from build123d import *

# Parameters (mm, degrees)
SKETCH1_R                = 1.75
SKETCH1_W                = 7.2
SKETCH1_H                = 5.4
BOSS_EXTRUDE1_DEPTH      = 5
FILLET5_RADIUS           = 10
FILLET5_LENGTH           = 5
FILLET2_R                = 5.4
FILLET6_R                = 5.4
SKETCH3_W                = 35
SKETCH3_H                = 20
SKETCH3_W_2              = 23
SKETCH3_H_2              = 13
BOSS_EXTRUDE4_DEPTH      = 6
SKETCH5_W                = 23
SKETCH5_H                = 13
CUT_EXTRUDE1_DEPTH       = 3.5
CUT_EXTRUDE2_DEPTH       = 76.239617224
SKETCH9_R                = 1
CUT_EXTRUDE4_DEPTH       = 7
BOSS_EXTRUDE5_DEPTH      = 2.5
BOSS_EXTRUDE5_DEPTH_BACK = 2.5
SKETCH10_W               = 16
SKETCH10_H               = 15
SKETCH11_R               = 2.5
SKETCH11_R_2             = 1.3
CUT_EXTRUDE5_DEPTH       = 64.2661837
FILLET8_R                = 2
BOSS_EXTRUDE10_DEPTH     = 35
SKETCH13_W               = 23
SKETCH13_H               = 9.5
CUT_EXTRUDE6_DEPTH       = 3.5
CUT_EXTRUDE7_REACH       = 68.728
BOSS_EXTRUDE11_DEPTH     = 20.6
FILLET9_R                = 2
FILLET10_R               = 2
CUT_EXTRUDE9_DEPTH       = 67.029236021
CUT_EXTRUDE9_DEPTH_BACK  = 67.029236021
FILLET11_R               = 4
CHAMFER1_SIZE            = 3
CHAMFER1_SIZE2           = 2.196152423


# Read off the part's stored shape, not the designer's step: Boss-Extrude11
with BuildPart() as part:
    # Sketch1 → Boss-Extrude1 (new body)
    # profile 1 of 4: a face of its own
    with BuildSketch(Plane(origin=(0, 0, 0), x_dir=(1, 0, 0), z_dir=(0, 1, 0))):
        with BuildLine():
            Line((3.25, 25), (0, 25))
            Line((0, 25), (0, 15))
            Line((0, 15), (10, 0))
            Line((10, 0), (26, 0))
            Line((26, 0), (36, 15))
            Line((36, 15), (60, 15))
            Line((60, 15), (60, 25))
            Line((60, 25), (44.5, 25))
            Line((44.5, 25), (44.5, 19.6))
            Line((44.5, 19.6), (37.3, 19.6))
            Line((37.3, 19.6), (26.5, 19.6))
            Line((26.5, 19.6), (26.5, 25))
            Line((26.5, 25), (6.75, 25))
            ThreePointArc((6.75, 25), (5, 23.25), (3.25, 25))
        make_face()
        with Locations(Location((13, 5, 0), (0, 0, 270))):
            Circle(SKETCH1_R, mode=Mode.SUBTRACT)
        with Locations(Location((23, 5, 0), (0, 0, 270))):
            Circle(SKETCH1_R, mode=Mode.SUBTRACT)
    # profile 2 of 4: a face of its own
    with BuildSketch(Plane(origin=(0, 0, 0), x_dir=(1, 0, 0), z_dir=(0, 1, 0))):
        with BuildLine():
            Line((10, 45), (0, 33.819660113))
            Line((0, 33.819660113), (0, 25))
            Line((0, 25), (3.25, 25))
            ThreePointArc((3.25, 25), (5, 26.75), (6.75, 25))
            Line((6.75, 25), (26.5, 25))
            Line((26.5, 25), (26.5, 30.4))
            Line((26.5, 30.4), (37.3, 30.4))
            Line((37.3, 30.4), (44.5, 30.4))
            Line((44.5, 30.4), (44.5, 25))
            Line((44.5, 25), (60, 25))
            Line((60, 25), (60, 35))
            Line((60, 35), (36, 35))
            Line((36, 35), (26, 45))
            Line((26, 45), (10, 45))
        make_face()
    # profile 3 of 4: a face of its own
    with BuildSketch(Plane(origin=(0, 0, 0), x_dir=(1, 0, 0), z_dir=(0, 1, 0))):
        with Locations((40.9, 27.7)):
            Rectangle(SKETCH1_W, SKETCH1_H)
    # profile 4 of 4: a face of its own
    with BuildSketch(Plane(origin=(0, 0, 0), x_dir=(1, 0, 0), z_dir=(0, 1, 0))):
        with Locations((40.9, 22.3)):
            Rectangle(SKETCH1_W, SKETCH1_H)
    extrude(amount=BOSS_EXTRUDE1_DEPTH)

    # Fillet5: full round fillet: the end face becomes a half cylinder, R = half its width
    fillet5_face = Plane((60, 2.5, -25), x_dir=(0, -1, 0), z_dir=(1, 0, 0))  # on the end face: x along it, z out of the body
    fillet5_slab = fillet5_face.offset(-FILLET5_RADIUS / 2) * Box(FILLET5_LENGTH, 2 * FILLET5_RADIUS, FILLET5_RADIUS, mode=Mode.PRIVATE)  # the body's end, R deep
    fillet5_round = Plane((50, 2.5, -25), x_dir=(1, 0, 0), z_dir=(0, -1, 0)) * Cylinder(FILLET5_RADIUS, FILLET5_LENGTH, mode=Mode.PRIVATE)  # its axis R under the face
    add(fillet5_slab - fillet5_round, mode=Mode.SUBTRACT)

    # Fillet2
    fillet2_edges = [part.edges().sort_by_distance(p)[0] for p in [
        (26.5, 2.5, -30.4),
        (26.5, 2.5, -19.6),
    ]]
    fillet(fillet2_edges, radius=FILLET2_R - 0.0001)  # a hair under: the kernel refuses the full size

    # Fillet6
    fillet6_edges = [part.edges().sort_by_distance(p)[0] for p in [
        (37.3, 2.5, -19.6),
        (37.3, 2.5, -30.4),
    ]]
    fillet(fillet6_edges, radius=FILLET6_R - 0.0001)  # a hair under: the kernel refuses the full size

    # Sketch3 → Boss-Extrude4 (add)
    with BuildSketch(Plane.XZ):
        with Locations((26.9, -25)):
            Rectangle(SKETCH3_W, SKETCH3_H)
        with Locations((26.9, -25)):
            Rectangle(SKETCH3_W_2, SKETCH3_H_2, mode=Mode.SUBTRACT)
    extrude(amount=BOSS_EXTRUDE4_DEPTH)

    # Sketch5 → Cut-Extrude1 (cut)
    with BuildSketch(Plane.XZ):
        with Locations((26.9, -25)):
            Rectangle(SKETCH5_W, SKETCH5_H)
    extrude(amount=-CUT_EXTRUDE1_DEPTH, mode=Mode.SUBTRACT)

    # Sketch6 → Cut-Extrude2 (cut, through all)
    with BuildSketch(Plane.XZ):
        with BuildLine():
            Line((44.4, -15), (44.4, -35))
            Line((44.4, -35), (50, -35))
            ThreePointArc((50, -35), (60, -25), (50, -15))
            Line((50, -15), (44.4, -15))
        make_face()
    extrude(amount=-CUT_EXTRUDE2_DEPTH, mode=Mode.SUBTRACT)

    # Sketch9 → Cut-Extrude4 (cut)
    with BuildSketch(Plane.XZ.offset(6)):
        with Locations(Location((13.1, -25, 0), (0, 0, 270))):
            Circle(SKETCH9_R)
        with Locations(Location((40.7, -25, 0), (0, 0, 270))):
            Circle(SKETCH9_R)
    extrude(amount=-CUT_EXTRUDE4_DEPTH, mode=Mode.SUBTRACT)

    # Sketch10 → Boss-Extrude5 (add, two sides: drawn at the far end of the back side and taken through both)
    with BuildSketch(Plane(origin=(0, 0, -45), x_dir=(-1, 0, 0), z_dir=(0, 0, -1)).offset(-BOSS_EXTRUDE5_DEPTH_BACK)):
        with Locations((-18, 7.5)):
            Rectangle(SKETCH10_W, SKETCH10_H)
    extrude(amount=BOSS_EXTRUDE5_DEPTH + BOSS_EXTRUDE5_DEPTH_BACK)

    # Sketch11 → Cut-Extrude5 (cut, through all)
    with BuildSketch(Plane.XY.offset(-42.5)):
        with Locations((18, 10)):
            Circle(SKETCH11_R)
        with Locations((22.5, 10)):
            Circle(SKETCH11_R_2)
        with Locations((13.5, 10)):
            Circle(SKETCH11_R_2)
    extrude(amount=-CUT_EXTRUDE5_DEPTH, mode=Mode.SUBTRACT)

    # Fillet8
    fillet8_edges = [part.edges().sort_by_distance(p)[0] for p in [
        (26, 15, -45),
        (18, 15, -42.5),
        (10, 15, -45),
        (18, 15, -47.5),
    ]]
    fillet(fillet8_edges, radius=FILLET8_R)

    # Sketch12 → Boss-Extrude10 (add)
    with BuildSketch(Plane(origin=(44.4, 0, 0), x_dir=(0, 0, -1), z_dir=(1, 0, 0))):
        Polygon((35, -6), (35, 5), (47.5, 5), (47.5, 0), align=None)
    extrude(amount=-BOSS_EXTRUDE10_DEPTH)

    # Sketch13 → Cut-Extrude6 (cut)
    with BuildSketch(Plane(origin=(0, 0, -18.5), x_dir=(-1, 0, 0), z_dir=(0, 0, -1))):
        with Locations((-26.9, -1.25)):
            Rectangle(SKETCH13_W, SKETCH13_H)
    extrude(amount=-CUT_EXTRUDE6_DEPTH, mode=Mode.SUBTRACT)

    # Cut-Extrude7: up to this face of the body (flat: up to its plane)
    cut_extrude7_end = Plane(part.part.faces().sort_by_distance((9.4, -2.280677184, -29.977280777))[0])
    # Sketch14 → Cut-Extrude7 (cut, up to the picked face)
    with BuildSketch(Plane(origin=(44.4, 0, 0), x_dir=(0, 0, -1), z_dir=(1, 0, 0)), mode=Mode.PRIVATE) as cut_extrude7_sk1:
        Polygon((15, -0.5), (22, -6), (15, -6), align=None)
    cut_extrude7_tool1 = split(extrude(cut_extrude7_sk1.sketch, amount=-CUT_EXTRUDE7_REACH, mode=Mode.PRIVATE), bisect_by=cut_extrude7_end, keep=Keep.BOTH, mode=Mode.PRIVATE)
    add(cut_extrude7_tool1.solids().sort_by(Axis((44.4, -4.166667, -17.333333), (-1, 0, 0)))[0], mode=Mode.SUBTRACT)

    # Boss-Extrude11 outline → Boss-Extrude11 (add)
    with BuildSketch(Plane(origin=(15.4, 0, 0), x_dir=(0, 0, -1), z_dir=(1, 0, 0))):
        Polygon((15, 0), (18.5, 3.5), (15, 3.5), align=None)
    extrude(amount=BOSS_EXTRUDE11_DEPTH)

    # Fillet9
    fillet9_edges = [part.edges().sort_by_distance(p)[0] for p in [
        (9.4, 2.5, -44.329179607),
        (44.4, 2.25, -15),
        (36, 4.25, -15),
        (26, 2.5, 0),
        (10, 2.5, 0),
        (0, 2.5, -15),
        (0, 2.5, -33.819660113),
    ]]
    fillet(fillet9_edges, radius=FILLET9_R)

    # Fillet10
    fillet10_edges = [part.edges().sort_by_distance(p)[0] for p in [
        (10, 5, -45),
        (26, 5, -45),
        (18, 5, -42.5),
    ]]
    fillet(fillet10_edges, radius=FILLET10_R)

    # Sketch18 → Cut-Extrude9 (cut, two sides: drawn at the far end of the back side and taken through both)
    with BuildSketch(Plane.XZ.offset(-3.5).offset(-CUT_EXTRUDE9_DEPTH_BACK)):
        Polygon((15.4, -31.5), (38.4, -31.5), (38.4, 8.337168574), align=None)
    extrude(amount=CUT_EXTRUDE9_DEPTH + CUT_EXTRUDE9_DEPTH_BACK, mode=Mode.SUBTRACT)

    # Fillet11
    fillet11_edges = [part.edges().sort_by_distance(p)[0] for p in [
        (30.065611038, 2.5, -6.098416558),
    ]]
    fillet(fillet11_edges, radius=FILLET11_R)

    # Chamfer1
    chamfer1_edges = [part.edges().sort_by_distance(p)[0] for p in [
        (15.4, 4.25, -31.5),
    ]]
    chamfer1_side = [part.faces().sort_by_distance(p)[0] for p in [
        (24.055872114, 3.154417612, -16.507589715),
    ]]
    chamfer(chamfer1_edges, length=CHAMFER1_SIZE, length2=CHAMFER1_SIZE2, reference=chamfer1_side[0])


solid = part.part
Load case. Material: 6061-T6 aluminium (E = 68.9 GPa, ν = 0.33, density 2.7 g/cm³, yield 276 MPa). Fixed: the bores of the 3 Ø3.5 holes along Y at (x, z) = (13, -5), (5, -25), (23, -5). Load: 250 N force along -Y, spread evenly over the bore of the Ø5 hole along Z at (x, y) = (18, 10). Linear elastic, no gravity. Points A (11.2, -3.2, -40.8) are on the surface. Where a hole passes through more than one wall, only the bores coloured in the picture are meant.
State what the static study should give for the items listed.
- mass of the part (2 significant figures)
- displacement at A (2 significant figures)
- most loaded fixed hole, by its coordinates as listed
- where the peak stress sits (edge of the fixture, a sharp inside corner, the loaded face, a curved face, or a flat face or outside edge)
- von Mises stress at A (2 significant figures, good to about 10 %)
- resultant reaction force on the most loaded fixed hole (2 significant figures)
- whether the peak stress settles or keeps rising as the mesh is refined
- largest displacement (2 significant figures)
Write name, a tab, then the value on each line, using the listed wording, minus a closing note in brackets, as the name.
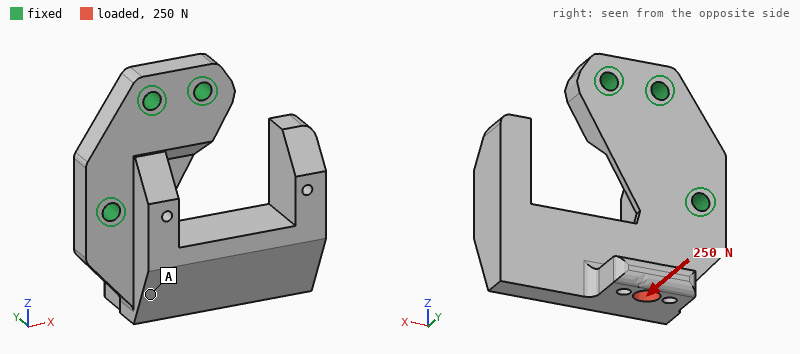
mass of the part	28 g
displacement at A	0.033 mm
most loaded fixed hole, by its coordinates as listed	(5, -25)
where the peak stress sits	edge of the fixture
von Mises stress at A	8.5 MPa
resultant reaction force on the most loaded fixed hole	370 N
whether the peak stress settles or keeps rising as the mesh is refined	keeps rising
largest displacement	0.10 mm
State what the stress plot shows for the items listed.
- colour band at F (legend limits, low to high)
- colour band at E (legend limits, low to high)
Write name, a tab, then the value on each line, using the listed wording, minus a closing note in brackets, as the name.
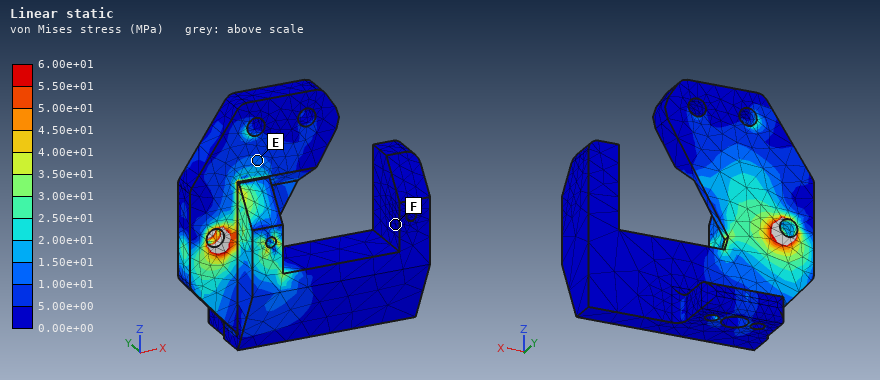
colour band at F	0.00e+00 to 5.00e+00 MPa
colour band at E	1.00e+01 to 1.50e+01 MPa
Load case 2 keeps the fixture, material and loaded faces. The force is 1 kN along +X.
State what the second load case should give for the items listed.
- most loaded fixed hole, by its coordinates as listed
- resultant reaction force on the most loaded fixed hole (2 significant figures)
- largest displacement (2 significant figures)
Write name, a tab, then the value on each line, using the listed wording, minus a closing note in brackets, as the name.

most loaded fixed hole, by its coordinates as listed	(5, -25)
resultant reaction force on the most loaded fixed hole	1.5 kN
largest displacement	0.22 mm
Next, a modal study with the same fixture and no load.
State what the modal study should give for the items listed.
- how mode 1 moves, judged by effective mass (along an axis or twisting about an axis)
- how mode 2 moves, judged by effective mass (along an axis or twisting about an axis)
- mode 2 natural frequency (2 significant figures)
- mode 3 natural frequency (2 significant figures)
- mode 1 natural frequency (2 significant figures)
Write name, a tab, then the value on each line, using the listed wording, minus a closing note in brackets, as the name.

how mode 1 moves, judged by effective mass	along Y
how mode 2 moves, judged by effective mass	along Z
mode 2 natural frequency	3600 Hz
mode 3 natural frequency	5400 Hz
mode 1 natural frequency	1900 Hz
